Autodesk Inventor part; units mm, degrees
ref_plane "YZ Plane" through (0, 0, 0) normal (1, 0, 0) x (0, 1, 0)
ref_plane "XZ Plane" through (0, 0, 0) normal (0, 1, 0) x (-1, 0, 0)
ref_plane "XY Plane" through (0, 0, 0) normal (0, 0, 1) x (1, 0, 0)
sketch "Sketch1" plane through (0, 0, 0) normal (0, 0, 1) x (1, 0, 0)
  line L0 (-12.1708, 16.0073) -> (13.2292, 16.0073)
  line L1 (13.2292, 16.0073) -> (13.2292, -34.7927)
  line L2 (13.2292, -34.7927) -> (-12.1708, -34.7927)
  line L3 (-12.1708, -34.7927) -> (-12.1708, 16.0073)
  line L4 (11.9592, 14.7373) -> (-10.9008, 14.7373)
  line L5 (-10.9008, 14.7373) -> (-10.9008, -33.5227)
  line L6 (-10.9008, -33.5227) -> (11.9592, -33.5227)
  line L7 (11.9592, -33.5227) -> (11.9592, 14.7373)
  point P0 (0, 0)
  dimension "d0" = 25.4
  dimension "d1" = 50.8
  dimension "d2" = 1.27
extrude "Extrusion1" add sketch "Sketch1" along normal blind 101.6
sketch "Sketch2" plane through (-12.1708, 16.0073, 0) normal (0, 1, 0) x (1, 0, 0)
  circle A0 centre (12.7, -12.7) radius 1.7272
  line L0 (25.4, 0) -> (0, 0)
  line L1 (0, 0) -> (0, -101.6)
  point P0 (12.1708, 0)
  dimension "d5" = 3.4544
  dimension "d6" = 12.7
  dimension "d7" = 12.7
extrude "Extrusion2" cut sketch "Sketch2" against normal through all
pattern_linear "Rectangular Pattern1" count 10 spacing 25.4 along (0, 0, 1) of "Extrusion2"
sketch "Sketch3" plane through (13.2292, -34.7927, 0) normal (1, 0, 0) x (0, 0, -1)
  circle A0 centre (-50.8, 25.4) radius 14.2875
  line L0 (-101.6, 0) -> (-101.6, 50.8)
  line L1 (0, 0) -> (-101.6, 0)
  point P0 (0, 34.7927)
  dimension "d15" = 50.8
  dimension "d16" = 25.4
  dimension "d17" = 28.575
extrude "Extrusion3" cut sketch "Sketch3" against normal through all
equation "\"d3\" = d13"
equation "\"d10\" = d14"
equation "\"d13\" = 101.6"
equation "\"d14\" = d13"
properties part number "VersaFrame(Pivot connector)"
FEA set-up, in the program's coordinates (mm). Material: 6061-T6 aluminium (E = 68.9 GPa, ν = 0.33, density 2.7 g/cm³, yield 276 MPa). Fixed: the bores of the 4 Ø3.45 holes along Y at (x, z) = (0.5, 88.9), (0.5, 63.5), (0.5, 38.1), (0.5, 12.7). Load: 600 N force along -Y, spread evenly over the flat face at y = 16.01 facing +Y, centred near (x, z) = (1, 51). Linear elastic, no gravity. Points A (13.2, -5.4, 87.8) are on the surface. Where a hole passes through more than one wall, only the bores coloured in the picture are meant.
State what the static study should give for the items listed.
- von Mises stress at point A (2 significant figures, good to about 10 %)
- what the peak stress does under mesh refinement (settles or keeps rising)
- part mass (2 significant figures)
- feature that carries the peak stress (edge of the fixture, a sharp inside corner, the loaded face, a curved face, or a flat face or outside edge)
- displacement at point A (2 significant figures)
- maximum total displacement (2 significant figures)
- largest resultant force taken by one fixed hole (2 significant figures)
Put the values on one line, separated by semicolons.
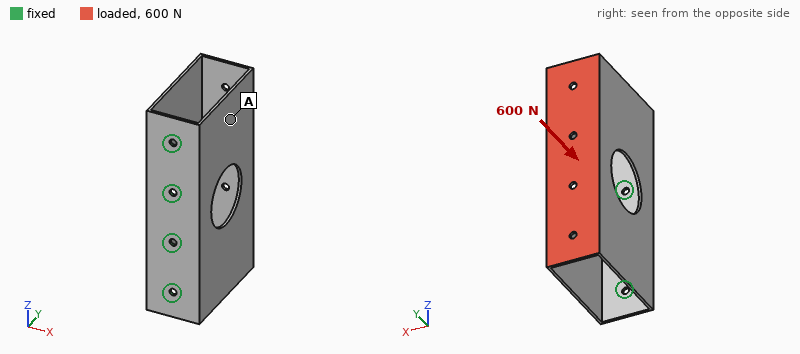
14 MPa; keeps rising; 47 g; edge of the fixture; 0.15 mm; 0.17 mm; 160 N
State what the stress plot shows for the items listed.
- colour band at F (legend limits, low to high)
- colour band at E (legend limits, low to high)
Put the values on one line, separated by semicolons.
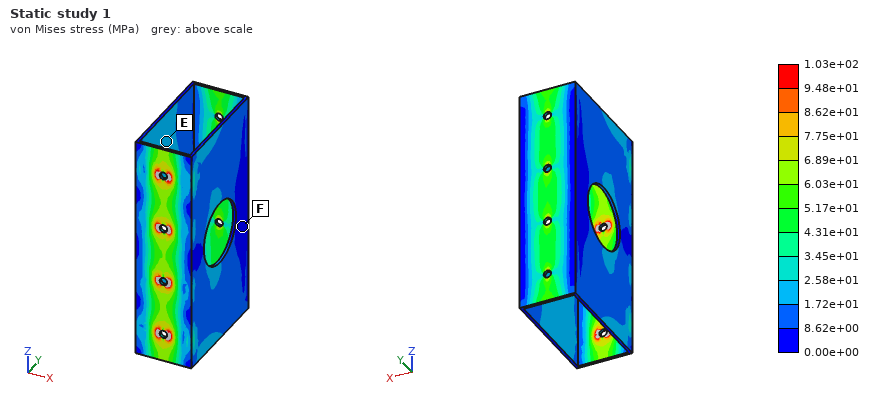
0.00e+00 to 8.62e+00 MPa; 1.72e+01 to 2.58e+01 MPa
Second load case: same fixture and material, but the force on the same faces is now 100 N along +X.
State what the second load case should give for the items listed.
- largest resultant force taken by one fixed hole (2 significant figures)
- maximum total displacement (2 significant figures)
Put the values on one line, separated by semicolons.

29 N; 1.3 mm
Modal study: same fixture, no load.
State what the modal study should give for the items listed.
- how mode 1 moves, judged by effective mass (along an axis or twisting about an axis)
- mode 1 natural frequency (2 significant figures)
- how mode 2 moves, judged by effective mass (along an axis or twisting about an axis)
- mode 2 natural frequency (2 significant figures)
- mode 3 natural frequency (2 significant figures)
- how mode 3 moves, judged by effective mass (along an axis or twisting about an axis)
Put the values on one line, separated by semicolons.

along X; 310 Hz; twisting about Y; 1000 Hz; 1300 Hz; along Z
